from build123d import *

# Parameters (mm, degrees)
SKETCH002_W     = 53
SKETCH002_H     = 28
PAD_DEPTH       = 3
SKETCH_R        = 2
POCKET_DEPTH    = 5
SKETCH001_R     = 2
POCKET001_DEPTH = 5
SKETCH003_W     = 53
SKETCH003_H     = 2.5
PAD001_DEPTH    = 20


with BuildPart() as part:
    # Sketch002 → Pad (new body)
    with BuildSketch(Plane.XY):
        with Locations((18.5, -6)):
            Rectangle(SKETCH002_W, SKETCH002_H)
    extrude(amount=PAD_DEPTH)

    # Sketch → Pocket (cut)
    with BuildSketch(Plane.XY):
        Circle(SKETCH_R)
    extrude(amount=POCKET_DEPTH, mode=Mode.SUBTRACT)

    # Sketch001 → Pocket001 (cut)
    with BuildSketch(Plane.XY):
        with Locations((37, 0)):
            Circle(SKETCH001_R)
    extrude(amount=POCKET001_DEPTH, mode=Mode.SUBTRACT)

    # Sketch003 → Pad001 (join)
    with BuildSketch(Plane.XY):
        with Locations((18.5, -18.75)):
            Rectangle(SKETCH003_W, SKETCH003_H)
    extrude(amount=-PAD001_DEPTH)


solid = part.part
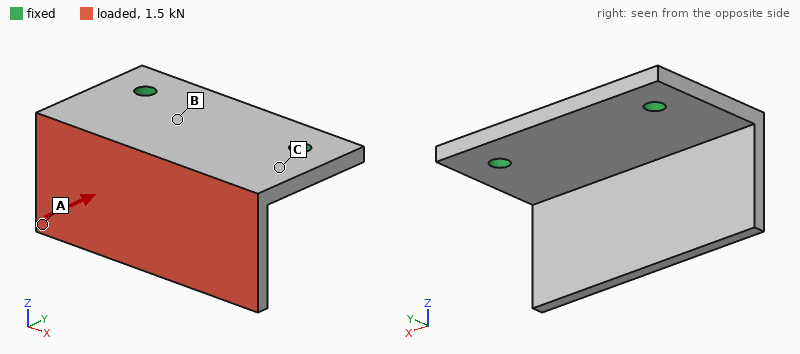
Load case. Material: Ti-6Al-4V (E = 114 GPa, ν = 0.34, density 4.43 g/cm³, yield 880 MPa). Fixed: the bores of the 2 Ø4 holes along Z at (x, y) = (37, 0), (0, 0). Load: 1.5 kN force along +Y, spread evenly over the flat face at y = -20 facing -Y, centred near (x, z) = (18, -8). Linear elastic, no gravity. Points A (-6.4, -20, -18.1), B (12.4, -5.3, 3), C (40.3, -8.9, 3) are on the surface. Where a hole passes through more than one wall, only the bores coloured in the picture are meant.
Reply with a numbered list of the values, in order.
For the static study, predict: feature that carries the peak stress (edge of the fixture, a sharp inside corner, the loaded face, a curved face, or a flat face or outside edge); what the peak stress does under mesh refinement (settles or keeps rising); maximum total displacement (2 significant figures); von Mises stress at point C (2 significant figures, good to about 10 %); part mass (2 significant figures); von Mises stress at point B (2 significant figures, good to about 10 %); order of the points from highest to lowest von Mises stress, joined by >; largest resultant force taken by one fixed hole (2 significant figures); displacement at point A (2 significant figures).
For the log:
1. edge of the fixture
2. keeps rising
3. 0.66 mm
4. 180 MPa
5. 31 g
6. 120 MPa
7. C > B > A
8. 770 N
9. 0.60 mm
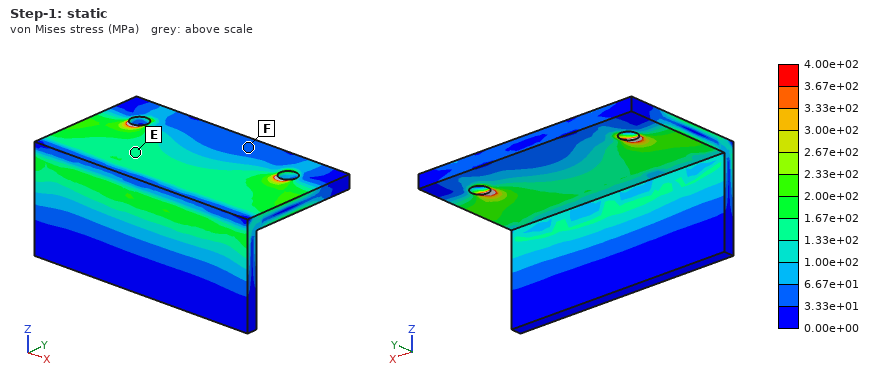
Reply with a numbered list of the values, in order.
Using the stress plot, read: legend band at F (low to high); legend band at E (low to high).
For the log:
1. 3.33e+01 to 6.67e+01 MPa
2. 1.33e+02 to 1.67e+02 MPa
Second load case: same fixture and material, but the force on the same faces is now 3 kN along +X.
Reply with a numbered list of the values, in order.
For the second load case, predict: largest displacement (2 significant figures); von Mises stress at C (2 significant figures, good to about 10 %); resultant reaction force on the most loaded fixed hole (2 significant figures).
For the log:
1. 0.31 mm
2. 140 MPa
3. 2.3 kN
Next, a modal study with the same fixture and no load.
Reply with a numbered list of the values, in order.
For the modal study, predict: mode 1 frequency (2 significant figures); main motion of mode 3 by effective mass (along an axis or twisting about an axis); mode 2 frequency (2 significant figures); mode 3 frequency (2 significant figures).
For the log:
1. 2100 Hz
2. along Z
3. 3500 Hz
4. 5100 Hz
